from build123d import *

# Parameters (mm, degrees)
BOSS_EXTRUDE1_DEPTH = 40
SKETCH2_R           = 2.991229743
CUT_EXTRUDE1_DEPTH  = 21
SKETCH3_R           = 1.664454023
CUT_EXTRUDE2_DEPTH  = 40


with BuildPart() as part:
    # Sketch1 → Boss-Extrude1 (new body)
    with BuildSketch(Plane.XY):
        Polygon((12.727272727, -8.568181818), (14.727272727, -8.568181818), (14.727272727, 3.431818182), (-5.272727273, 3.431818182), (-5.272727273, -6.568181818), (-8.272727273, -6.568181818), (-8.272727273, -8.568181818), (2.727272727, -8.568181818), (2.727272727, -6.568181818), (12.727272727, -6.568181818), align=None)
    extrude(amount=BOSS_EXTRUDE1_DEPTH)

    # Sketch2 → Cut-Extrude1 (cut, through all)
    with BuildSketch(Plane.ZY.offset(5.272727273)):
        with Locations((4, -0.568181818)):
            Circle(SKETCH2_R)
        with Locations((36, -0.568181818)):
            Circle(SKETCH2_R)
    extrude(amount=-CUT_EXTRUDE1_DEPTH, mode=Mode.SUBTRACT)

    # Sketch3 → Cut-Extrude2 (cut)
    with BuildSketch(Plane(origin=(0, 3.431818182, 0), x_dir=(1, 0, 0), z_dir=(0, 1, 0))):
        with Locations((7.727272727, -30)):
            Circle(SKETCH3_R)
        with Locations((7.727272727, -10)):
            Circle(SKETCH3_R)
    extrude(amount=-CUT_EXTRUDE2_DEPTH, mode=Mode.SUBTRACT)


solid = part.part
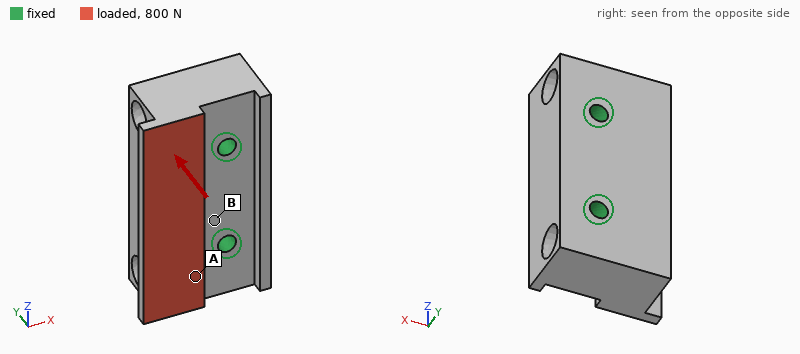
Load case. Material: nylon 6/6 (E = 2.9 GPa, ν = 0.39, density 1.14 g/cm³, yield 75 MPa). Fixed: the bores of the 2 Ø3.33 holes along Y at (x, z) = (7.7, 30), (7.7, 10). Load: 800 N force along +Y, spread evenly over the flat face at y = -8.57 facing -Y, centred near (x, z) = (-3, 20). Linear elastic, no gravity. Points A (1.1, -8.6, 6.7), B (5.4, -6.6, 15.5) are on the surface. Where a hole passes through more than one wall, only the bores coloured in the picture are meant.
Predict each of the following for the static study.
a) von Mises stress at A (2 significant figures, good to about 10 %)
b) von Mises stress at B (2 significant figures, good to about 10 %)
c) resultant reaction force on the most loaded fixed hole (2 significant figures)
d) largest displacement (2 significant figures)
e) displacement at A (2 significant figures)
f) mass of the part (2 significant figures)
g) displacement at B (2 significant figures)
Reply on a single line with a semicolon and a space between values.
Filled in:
3.4 MPa; 6.3 MPa; 400 N; 0.21 mm; 0.080 mm; 8.8 g; 0.034 mm
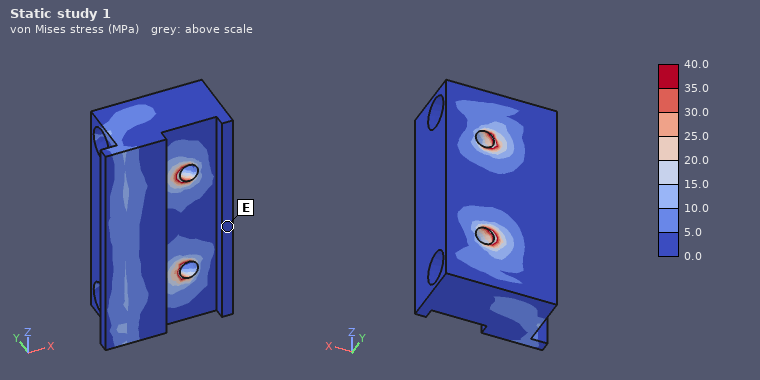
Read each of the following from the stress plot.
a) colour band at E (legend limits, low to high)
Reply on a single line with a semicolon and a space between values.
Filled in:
0.0 to 5.0 MPa
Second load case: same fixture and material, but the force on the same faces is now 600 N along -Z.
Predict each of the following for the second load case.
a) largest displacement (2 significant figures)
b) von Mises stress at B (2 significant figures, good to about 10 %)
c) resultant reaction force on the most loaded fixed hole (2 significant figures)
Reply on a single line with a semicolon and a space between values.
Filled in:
96 µm; 6.6 MPa; 430 N
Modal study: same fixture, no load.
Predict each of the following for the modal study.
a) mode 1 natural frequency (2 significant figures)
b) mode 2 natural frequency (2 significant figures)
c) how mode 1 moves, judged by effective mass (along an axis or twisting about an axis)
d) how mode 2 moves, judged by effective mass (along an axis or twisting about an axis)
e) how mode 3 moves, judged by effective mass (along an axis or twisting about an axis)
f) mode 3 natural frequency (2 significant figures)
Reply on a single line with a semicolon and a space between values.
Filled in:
7300 Hz; 8600 Hz; along Y; twisting about X; along Z; 11 kHz
